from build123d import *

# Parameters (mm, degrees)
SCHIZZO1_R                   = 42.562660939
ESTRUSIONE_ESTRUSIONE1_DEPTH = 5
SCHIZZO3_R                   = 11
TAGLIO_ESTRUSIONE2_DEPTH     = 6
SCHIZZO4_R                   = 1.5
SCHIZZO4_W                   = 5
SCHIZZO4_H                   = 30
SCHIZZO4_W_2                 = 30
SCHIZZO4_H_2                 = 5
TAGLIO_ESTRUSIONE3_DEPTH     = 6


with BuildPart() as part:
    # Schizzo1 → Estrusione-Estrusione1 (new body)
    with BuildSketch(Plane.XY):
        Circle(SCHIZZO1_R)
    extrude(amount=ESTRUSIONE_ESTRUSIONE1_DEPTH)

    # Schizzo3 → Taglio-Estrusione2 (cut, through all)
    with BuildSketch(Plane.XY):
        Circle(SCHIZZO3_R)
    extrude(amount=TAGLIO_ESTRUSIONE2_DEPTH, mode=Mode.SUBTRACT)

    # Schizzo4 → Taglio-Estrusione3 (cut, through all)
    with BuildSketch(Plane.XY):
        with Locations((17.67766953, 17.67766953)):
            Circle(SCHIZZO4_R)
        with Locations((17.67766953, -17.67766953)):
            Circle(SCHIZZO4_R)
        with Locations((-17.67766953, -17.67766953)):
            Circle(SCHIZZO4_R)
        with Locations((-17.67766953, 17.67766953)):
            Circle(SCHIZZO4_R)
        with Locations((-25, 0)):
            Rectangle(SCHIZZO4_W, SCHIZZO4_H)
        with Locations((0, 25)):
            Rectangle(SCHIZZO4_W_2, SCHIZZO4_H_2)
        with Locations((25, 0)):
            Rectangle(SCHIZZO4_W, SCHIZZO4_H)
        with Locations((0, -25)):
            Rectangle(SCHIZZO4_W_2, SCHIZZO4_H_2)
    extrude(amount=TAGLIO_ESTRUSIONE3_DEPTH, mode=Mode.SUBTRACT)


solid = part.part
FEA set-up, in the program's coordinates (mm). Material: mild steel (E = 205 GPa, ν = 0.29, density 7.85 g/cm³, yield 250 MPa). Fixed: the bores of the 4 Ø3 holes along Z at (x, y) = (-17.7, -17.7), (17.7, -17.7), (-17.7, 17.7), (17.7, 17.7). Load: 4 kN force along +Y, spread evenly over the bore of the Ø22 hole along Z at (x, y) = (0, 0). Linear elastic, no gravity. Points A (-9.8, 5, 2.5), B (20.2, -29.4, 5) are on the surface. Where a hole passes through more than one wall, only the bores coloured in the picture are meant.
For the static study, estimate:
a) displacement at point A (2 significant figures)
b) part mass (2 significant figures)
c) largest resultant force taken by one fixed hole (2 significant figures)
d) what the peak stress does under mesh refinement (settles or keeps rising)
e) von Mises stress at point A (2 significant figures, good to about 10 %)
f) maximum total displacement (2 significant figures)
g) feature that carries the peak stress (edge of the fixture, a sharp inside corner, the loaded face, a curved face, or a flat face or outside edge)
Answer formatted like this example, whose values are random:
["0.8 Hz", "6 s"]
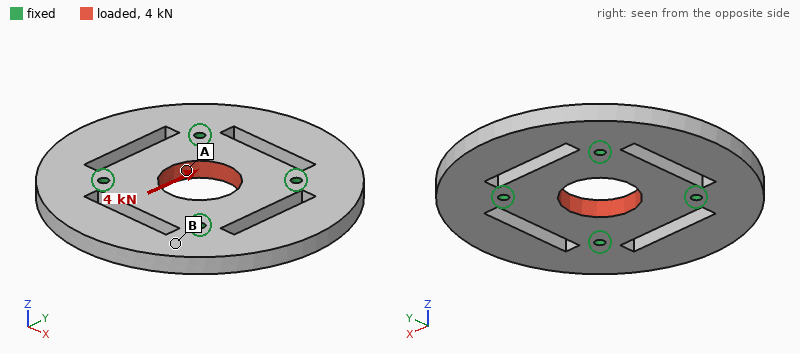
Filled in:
["1.5 µm", "180 g", "1.0 kN", "keeps rising", "25 MPa", "2.6 µm", "edge of the fixture"]
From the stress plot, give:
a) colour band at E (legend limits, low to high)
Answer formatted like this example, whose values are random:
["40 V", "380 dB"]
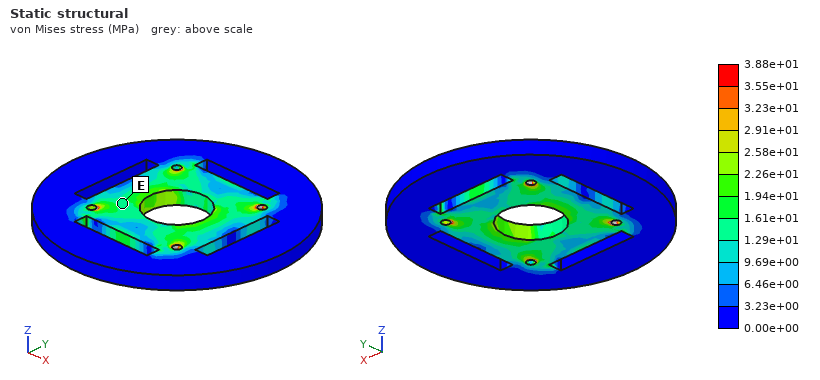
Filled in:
["1.29e+01 to 1.61e+01 MPa"]
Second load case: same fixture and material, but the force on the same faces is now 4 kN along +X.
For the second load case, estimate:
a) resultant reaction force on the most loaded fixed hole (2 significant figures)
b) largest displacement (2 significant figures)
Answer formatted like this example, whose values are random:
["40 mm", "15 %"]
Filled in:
["1.0 kN", "2.6 µm"]
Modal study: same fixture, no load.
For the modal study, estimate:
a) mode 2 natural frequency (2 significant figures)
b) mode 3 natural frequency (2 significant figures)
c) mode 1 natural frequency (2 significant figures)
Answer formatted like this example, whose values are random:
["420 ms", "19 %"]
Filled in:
["5400 Hz", "5400 Hz", "4700 Hz"]
